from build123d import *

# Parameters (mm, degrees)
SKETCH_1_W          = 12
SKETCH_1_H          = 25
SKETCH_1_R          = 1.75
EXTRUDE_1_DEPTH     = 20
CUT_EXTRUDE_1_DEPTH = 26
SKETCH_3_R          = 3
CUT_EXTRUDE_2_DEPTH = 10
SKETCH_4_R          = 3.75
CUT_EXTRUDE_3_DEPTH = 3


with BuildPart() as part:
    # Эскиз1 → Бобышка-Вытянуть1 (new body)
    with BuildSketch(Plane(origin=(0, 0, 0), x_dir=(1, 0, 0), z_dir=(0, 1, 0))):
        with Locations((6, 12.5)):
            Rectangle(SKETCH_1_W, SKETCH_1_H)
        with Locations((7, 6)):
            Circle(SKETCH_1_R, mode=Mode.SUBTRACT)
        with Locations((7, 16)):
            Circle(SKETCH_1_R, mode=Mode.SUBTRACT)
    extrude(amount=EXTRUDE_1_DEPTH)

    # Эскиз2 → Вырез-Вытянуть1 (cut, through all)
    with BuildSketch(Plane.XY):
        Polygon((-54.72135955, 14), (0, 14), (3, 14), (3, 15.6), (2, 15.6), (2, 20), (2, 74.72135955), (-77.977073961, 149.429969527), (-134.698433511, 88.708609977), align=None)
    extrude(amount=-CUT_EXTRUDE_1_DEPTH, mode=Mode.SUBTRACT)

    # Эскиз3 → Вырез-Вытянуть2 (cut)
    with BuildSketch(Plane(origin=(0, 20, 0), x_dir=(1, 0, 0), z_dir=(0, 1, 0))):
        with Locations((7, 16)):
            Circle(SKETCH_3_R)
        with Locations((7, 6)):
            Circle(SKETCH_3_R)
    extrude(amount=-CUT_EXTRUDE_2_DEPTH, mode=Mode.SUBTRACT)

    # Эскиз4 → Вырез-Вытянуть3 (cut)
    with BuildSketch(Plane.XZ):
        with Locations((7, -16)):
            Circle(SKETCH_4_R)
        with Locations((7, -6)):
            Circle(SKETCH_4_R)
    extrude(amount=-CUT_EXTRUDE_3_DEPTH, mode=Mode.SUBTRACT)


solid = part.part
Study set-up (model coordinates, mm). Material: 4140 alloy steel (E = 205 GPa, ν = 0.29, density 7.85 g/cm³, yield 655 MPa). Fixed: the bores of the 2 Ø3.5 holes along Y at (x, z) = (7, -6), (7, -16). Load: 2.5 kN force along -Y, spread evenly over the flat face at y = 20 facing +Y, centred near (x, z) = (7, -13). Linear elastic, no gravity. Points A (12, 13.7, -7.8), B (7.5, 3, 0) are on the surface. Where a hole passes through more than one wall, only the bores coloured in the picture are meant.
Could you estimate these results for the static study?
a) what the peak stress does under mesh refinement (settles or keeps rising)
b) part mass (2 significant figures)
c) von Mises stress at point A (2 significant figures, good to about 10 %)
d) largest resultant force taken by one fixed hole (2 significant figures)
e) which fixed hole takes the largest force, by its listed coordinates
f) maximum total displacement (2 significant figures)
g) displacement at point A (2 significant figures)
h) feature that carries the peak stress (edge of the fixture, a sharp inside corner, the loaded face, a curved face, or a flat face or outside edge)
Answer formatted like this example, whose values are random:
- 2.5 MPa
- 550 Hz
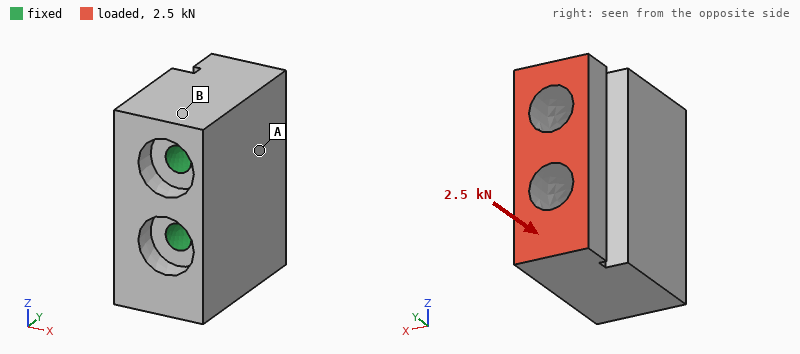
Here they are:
- keeps rising
- 37 g
- 12 MPa
- 1.6 kN
- (7, -16)
- 2.2 µm
- 0.62 µm
- edge of the fixture
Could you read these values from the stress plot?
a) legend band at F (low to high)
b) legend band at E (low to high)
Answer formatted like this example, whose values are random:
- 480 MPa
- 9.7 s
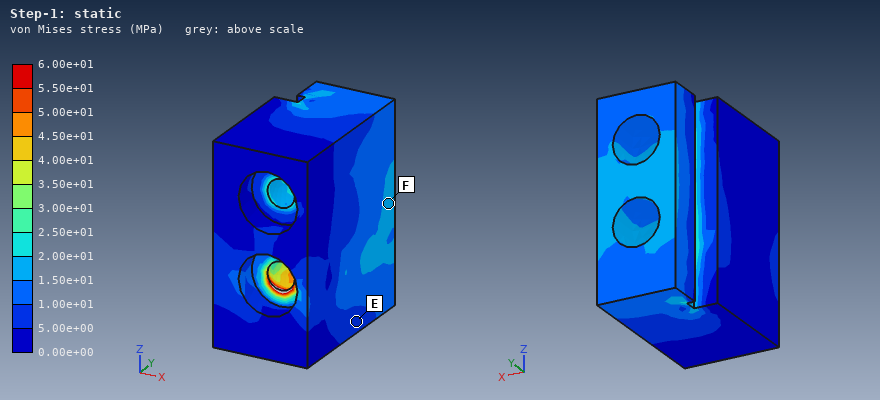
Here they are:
- 1.50e+01 to 2.00e+01 MPa
- 5.00e+00 to 1.00e+01 MPa
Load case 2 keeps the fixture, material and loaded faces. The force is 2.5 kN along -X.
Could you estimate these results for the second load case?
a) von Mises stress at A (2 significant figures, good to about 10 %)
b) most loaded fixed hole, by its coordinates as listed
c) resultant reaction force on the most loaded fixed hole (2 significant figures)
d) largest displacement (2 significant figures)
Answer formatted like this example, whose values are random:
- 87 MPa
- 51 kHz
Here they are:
- 41 MPa
- (7, -16)
- 1.6 kN
- 15 µm
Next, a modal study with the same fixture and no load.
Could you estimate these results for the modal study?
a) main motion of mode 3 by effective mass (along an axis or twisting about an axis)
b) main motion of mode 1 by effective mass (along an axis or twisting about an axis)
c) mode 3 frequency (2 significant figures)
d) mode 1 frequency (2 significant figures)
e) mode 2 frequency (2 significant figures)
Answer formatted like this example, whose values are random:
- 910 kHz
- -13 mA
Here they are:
- twisting about Y
- along X
- 35 kHz
- 26 kHz
- 32 kHz
